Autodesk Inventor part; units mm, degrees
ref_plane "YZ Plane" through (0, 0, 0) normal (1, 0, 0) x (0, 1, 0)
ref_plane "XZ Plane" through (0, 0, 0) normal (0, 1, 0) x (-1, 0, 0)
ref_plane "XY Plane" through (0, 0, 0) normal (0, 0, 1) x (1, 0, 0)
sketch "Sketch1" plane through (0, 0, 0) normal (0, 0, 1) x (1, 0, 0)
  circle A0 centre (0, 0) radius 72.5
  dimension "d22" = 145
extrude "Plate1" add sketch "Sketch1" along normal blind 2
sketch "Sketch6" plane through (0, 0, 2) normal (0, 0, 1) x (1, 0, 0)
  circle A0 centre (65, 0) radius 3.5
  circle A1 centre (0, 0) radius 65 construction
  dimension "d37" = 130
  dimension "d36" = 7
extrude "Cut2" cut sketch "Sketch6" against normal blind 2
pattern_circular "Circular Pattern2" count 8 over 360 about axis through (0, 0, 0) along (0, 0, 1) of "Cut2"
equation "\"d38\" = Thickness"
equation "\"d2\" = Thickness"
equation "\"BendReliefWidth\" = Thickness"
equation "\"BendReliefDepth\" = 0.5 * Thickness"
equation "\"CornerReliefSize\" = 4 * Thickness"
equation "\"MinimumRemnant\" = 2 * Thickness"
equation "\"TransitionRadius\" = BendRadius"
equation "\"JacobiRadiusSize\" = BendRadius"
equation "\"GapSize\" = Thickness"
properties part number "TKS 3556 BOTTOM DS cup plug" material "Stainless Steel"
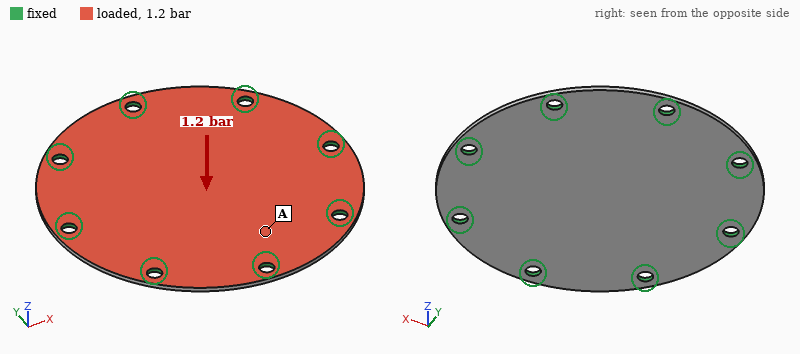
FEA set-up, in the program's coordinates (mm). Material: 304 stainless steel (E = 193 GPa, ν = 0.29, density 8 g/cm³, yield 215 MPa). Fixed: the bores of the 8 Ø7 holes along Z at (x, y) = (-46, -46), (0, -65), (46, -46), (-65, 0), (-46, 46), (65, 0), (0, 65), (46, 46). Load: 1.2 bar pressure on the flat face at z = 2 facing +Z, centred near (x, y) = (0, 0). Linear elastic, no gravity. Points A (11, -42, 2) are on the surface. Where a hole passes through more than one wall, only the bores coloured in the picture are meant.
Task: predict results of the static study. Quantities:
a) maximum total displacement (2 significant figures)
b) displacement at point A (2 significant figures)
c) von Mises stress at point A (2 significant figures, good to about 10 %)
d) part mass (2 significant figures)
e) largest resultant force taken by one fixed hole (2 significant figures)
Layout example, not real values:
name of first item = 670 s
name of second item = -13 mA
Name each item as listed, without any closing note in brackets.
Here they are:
maximum total displacement = 0.26 mm
displacement at point A = 0.088 mm
von Mises stress at point A = 35 MPa
part mass = 260 g
largest resultant force taken by one fixed hole = 240 N
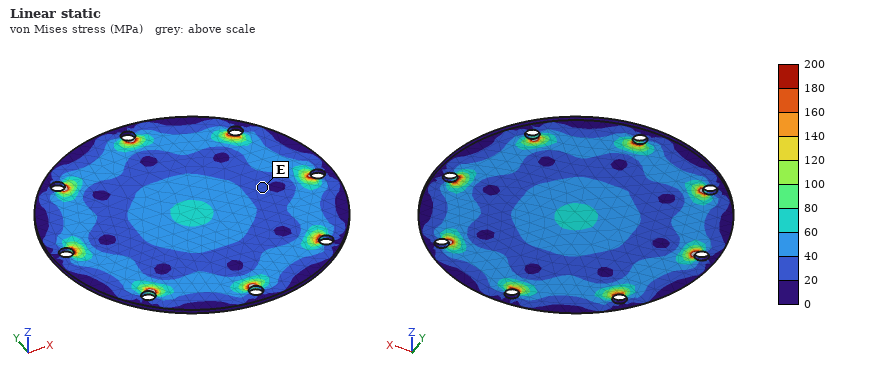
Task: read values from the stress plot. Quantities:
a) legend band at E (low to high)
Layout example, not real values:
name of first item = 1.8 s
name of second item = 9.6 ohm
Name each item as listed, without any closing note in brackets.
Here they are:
legend band at E = 20 to 40 MPa
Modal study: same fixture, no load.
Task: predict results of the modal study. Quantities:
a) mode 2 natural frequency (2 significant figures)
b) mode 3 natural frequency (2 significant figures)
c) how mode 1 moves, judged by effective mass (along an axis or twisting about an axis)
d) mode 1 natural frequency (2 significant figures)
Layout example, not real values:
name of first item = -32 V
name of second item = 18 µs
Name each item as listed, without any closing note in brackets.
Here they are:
mode 2 natural frequency = 2200 Hz
mode 3 natural frequency = 2200 Hz
how mode 1 moves, judged by effective mass = along Z
mode 1 natural frequency = 1100 Hz
